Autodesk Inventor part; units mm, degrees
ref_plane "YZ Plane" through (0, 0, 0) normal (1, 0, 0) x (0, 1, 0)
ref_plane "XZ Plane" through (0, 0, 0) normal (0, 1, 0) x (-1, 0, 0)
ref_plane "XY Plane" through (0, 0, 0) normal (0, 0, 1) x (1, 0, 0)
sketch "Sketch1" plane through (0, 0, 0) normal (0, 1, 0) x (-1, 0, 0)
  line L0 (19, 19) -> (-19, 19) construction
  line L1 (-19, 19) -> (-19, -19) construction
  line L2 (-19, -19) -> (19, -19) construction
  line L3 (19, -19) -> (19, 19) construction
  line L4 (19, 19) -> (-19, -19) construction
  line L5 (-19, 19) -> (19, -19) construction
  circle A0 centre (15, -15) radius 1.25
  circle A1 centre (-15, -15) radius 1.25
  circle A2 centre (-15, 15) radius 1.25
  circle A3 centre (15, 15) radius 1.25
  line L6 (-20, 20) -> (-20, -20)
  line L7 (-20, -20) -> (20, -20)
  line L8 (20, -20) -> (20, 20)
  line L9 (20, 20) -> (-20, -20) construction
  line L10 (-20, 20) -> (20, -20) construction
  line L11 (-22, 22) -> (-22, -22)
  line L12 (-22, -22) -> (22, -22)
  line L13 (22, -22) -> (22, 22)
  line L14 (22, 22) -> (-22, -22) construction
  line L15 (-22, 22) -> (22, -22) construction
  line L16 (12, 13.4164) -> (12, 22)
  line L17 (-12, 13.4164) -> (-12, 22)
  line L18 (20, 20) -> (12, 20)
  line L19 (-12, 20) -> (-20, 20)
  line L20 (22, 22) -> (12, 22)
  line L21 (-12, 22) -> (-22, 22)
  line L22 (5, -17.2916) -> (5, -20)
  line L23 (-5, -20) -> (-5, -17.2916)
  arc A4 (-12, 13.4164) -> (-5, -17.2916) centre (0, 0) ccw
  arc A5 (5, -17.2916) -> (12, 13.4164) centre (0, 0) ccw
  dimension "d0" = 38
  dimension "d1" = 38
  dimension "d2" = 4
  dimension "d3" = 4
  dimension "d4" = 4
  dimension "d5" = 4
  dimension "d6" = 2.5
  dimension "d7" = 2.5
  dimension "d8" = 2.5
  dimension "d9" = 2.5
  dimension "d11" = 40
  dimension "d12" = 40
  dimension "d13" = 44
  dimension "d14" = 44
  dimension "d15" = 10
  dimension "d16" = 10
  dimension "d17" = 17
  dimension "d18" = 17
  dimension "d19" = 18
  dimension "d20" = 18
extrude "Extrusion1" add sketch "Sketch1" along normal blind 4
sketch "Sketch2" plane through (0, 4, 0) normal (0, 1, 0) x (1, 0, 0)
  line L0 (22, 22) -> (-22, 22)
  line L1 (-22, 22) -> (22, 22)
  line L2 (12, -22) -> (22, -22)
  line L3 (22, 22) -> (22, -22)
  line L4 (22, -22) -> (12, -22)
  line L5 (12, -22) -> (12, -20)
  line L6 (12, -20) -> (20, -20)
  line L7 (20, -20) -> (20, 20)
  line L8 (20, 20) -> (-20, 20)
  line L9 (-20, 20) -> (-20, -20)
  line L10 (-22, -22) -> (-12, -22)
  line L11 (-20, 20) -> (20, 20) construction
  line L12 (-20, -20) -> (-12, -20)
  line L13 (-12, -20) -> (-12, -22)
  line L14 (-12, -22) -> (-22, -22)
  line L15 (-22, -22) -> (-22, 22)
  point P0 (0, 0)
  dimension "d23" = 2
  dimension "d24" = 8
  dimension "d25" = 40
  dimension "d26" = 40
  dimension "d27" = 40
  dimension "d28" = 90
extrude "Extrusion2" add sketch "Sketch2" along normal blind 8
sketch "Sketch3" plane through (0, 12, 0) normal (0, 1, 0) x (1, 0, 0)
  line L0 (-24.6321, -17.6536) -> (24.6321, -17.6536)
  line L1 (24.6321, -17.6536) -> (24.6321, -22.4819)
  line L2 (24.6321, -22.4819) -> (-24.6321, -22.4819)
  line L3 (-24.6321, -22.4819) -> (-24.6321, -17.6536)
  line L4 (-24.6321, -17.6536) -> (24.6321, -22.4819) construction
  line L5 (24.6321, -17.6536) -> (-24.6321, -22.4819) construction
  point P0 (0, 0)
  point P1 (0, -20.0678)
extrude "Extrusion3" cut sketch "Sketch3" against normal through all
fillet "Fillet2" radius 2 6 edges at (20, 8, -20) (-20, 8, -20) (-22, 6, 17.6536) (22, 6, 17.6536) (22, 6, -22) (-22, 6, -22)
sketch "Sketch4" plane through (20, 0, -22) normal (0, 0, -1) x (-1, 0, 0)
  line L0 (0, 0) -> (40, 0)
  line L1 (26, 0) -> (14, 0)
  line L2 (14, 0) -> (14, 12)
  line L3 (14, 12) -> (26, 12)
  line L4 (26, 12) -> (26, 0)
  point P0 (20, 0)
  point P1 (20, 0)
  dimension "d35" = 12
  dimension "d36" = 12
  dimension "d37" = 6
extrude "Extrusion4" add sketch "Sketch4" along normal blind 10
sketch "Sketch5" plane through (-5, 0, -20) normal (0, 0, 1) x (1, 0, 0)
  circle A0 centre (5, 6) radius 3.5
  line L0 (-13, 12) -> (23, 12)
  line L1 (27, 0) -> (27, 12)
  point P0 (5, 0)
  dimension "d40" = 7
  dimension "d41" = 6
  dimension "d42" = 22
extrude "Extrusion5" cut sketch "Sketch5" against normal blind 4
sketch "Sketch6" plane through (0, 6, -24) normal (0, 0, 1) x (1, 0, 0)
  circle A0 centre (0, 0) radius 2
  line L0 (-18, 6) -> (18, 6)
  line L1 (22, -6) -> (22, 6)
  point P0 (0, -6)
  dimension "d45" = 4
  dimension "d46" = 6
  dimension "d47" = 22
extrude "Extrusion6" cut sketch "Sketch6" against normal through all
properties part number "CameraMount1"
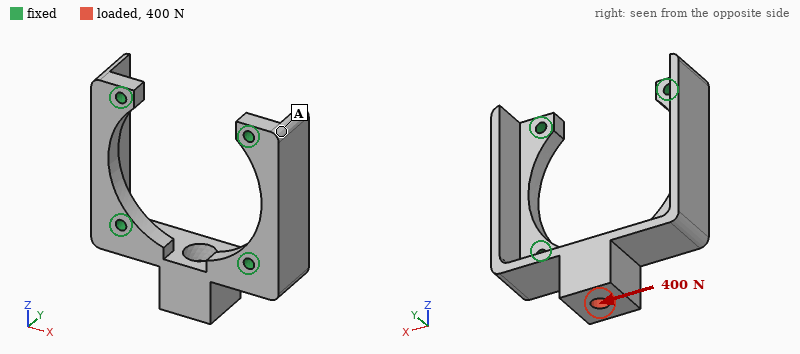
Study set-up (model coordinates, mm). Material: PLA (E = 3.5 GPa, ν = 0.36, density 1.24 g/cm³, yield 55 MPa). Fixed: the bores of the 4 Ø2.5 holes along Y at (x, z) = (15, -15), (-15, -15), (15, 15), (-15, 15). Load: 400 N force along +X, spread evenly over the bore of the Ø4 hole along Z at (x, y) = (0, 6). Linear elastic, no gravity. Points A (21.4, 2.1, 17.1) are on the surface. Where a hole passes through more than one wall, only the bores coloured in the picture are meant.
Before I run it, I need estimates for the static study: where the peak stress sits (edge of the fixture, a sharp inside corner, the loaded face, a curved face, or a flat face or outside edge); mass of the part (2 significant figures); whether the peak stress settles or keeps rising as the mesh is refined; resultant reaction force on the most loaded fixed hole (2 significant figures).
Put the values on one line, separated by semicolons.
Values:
edge of the fixture; 7.1 g; keeps rising; 280 N
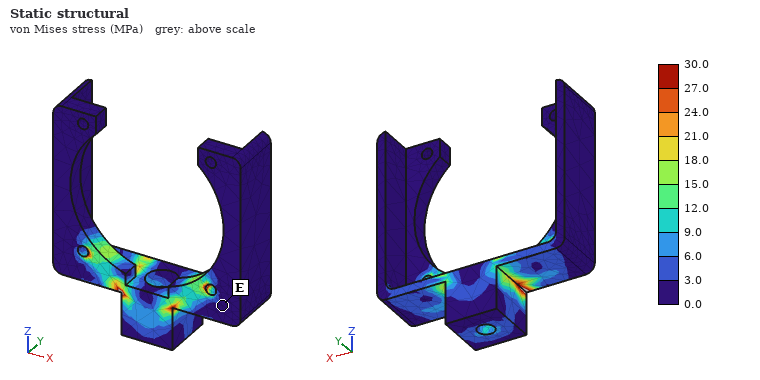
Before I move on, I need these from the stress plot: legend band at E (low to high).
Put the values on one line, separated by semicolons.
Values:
0.0 to 3.0 MPa
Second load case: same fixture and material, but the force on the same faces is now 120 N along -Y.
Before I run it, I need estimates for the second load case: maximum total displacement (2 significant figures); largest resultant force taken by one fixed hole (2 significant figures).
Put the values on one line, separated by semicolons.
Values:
0.67 mm; 76 N
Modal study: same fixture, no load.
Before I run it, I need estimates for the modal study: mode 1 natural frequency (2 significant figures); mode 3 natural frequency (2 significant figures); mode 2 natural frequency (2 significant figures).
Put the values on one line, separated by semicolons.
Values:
1900 Hz; 4500 Hz; 4500 Hz
